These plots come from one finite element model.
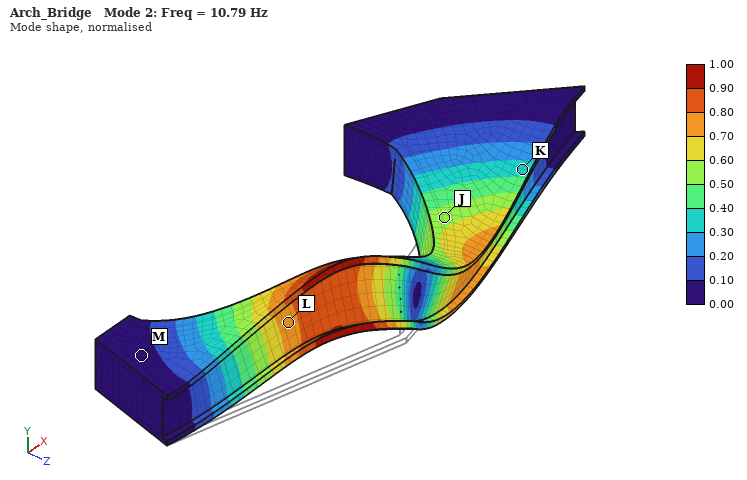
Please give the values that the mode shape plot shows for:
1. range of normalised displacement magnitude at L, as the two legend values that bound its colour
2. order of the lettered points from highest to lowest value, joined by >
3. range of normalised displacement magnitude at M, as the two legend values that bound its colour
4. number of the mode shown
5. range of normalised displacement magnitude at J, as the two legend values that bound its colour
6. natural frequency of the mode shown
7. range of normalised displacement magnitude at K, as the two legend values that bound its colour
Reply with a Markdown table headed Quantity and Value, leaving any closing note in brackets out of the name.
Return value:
| Quantity | Value |
|---|---|
| range of normalised displacement magnitude at L, as the two legend values that bound its colour | 0.70 to 0.80 |
| order of the lettered points from highest to lowest value, joined by > | L > J > K > M |
| range of normalised displacement magnitude at M, as the two legend values that bound its colour | 0.00 to 0.10 |
| number of the mode shown | 2 |
| range of normalised displacement magnitude at J, as the two legend values that bound its colour | 0.50 to 0.60 |
| natural frequency of the mode shown | 10.79 Hz |
| range of normalised displacement magnitude at K, as the two legend values that bound its colour | 0.30 to 0.40 |
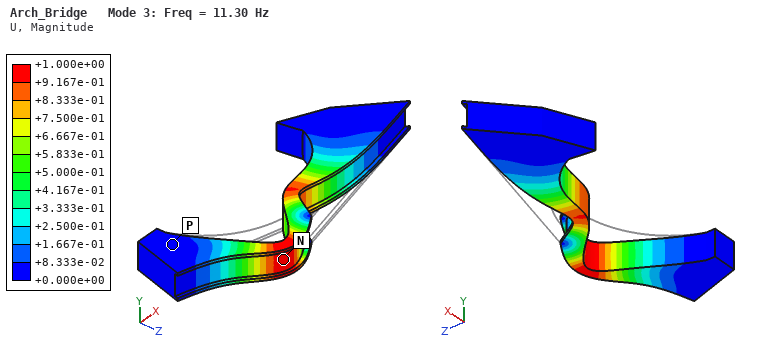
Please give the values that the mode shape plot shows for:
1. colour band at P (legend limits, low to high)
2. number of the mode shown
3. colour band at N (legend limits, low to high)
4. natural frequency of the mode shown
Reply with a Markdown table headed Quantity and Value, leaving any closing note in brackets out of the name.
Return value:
| Quantity | Value |
|---|---|
| colour band at P | +0.000e+00 to +8.333e-02 |
| number of the mode shown | 3 |
| colour band at N | +9.167e-01 to +1.000e+00 |
| natural frequency of the mode shown | 11.30 Hz |
